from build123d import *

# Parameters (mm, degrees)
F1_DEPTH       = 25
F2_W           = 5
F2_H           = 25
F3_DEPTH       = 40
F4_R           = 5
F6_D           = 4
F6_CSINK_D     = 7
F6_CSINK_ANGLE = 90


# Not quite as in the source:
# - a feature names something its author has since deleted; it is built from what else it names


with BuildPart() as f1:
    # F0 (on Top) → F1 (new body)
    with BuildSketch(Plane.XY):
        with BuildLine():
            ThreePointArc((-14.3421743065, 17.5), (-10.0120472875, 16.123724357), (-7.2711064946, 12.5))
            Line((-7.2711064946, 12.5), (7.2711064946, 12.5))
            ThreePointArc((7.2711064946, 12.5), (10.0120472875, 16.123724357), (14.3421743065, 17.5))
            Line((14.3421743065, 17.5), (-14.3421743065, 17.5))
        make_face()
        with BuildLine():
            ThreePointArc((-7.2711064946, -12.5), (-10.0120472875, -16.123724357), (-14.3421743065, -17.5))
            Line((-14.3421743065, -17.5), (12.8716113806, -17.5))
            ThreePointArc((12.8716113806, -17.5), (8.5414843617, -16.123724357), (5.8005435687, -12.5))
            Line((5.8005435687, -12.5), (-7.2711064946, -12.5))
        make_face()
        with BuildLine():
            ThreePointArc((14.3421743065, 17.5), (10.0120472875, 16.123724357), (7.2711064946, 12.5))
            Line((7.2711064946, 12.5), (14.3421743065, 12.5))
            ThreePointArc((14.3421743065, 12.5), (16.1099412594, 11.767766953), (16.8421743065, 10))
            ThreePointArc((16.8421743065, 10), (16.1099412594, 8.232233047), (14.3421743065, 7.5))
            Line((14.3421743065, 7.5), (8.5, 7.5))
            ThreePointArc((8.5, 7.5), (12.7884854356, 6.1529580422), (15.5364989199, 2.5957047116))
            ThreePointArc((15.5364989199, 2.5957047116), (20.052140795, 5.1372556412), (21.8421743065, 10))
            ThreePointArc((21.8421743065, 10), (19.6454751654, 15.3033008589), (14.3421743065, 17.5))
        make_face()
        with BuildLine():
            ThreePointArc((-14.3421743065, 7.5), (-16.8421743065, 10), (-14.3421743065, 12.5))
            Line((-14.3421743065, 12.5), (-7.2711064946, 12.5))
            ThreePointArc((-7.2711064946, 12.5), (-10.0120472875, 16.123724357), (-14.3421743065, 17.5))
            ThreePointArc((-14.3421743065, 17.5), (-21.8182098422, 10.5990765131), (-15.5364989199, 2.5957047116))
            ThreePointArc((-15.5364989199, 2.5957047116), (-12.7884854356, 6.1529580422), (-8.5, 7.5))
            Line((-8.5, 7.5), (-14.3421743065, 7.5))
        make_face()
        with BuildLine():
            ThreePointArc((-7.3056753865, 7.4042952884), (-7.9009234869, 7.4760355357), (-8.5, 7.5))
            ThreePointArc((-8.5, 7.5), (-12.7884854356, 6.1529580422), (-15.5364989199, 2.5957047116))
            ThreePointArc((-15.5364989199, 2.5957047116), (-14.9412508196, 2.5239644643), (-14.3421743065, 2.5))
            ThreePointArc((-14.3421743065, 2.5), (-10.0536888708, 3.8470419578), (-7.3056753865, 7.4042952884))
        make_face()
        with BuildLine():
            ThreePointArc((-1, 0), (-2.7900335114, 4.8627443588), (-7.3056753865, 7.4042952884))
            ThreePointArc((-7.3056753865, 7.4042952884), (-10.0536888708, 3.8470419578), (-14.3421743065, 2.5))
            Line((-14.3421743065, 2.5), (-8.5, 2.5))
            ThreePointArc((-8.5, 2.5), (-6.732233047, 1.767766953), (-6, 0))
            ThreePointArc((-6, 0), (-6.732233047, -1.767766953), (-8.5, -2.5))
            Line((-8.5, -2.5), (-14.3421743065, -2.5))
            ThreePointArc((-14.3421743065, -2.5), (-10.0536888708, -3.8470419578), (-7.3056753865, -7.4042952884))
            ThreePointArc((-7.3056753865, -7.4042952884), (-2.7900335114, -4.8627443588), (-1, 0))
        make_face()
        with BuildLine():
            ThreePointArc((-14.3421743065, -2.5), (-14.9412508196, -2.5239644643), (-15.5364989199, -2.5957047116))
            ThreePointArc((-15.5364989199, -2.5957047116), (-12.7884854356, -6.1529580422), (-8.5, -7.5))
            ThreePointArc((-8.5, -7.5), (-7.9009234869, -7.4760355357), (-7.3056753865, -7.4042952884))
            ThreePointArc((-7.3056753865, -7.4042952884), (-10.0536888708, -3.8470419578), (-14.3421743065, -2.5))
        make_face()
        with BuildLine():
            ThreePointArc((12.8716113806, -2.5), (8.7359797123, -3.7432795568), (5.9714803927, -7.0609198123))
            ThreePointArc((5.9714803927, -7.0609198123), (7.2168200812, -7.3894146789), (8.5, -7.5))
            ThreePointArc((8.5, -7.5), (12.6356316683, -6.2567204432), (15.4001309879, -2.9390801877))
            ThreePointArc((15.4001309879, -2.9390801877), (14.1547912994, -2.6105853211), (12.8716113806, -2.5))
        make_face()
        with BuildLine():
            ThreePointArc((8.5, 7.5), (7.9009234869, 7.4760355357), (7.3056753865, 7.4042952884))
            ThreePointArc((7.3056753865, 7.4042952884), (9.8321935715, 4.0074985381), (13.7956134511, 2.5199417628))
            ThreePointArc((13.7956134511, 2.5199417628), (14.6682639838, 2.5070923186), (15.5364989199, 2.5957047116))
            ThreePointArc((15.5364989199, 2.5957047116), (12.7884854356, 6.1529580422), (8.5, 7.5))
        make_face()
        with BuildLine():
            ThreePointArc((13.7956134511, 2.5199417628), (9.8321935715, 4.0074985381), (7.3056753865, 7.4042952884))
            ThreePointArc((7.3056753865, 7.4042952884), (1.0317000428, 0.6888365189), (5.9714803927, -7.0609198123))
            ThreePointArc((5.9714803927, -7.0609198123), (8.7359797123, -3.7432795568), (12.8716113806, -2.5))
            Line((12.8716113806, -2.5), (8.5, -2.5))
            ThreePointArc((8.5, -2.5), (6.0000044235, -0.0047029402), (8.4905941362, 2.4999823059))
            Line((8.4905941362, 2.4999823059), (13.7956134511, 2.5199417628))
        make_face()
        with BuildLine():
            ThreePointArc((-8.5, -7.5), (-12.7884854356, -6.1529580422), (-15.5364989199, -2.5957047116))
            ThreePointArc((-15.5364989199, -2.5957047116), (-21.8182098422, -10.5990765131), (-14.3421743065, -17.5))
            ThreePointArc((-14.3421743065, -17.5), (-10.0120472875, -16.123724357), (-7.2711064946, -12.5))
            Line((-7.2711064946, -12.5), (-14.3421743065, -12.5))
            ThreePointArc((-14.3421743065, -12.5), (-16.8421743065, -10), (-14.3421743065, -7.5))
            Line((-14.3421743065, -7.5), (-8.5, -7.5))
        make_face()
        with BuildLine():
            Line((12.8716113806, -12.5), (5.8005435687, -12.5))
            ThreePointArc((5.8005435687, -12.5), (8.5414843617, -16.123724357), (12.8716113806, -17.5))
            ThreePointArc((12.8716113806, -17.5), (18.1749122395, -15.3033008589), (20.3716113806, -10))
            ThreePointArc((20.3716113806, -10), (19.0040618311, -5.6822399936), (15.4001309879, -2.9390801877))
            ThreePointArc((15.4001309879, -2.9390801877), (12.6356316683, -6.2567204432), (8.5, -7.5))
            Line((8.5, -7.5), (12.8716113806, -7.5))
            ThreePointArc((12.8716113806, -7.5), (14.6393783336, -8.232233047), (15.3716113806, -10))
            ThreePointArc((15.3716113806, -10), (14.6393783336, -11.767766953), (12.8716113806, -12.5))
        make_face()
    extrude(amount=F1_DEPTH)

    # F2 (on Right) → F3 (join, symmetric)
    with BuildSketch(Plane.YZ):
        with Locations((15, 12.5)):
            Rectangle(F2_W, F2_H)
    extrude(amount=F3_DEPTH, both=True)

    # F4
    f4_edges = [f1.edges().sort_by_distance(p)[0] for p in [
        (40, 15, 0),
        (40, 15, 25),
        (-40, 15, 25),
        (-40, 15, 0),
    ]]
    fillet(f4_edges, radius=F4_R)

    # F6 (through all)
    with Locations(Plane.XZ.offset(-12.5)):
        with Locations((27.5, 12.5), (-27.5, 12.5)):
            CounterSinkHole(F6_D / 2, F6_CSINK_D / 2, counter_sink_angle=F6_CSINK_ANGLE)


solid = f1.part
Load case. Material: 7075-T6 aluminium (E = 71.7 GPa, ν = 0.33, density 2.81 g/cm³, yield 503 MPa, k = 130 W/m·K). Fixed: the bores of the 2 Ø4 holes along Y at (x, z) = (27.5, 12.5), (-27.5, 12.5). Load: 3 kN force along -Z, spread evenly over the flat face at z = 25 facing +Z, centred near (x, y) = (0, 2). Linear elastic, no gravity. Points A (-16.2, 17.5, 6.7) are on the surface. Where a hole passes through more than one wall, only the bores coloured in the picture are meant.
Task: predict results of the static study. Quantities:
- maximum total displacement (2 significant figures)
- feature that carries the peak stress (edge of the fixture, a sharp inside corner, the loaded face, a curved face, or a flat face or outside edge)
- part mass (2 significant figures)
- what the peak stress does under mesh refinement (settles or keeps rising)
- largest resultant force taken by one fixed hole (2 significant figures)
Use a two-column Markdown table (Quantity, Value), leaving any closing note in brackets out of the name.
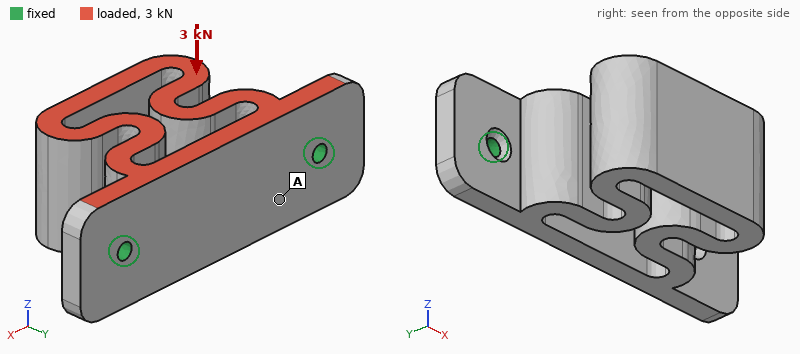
| Quantity | Value |
|---|---|
| maximum total displacement | 0.39 mm |
| feature that carries the peak stress | edge of the fixture |
| part mass | 74 g |
| what the peak stress does under mesh refinement | keeps rising |
| largest resultant force taken by one fixed hole | 1.5 kN |
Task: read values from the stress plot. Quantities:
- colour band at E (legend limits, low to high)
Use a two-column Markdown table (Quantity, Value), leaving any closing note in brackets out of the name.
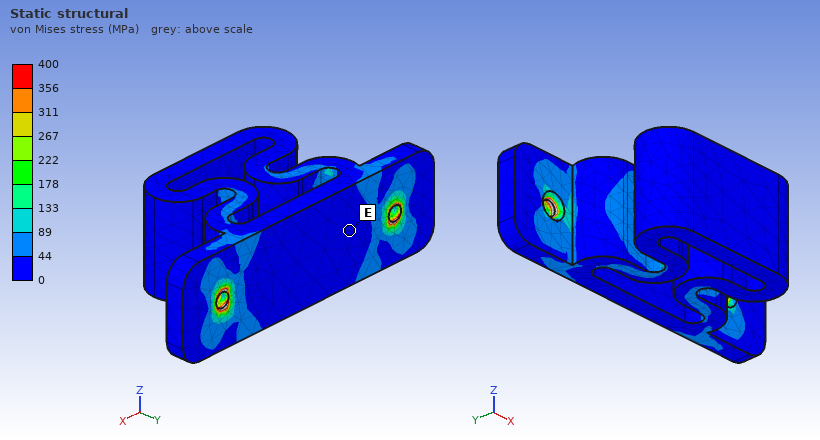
| Quantity | Value |
|---|---|
| colour band at E | 0 to 44 MPa |
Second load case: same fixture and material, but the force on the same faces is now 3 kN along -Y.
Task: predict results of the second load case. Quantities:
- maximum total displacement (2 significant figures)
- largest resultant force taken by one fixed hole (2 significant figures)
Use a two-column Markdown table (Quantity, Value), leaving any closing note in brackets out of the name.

| Quantity | Value |
|---|---|
| maximum total displacement | 0.43 mm |
| largest resultant force taken by one fixed hole | 1.7 kN |
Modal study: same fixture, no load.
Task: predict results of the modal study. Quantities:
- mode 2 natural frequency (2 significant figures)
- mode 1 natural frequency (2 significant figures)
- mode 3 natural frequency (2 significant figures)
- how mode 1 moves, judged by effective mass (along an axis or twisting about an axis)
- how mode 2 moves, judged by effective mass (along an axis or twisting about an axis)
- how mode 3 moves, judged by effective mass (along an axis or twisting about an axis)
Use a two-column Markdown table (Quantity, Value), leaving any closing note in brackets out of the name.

| Quantity | Value |
|---|---|
| mode 2 natural frequency | 2700 Hz |
| mode 1 natural frequency | 1900 Hz |
| mode 3 natural frequency | 3400 Hz |
| how mode 1 moves, judged by effective mass | along Z |
| how mode 2 moves, judged by effective mass | along X |
| how mode 3 moves, judged by effective mass | along Y |
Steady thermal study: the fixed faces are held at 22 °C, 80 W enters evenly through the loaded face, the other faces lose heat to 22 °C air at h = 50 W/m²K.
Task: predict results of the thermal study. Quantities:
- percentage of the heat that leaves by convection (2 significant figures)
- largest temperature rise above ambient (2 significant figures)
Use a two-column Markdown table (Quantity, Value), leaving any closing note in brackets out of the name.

| Quantity | Value |
|---|---|
| percentage of the heat that leaves by convection | 24 % |
| largest temperature rise above ambient | 59 K |
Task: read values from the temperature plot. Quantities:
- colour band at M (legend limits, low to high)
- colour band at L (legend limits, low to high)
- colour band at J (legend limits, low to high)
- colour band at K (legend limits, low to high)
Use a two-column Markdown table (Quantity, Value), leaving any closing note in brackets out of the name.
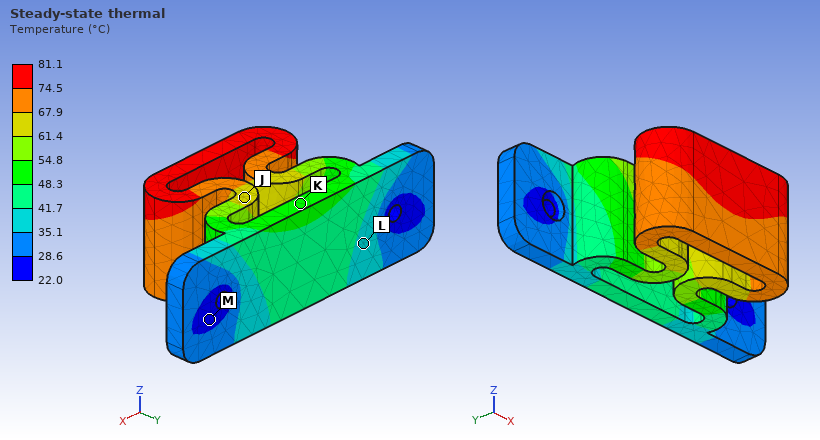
| Quantity | Value |
|---|---|
| colour band at M | 22.0 to 28.6 °C |
| colour band at L | 35.1 to 41.7 °C |
| colour band at J | 61.4 to 67.9 °C |
| colour band at K | 48.3 to 54.8 °C |
